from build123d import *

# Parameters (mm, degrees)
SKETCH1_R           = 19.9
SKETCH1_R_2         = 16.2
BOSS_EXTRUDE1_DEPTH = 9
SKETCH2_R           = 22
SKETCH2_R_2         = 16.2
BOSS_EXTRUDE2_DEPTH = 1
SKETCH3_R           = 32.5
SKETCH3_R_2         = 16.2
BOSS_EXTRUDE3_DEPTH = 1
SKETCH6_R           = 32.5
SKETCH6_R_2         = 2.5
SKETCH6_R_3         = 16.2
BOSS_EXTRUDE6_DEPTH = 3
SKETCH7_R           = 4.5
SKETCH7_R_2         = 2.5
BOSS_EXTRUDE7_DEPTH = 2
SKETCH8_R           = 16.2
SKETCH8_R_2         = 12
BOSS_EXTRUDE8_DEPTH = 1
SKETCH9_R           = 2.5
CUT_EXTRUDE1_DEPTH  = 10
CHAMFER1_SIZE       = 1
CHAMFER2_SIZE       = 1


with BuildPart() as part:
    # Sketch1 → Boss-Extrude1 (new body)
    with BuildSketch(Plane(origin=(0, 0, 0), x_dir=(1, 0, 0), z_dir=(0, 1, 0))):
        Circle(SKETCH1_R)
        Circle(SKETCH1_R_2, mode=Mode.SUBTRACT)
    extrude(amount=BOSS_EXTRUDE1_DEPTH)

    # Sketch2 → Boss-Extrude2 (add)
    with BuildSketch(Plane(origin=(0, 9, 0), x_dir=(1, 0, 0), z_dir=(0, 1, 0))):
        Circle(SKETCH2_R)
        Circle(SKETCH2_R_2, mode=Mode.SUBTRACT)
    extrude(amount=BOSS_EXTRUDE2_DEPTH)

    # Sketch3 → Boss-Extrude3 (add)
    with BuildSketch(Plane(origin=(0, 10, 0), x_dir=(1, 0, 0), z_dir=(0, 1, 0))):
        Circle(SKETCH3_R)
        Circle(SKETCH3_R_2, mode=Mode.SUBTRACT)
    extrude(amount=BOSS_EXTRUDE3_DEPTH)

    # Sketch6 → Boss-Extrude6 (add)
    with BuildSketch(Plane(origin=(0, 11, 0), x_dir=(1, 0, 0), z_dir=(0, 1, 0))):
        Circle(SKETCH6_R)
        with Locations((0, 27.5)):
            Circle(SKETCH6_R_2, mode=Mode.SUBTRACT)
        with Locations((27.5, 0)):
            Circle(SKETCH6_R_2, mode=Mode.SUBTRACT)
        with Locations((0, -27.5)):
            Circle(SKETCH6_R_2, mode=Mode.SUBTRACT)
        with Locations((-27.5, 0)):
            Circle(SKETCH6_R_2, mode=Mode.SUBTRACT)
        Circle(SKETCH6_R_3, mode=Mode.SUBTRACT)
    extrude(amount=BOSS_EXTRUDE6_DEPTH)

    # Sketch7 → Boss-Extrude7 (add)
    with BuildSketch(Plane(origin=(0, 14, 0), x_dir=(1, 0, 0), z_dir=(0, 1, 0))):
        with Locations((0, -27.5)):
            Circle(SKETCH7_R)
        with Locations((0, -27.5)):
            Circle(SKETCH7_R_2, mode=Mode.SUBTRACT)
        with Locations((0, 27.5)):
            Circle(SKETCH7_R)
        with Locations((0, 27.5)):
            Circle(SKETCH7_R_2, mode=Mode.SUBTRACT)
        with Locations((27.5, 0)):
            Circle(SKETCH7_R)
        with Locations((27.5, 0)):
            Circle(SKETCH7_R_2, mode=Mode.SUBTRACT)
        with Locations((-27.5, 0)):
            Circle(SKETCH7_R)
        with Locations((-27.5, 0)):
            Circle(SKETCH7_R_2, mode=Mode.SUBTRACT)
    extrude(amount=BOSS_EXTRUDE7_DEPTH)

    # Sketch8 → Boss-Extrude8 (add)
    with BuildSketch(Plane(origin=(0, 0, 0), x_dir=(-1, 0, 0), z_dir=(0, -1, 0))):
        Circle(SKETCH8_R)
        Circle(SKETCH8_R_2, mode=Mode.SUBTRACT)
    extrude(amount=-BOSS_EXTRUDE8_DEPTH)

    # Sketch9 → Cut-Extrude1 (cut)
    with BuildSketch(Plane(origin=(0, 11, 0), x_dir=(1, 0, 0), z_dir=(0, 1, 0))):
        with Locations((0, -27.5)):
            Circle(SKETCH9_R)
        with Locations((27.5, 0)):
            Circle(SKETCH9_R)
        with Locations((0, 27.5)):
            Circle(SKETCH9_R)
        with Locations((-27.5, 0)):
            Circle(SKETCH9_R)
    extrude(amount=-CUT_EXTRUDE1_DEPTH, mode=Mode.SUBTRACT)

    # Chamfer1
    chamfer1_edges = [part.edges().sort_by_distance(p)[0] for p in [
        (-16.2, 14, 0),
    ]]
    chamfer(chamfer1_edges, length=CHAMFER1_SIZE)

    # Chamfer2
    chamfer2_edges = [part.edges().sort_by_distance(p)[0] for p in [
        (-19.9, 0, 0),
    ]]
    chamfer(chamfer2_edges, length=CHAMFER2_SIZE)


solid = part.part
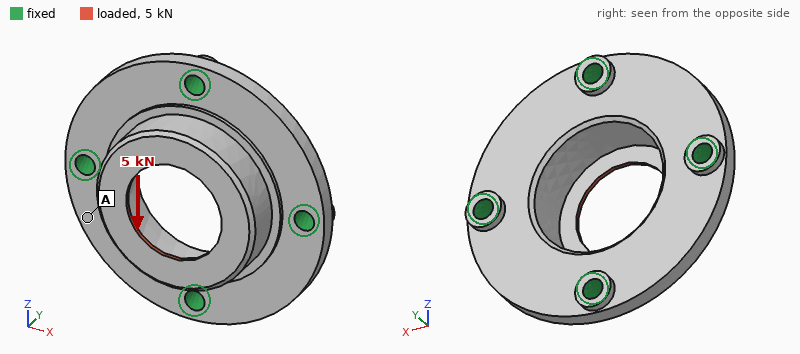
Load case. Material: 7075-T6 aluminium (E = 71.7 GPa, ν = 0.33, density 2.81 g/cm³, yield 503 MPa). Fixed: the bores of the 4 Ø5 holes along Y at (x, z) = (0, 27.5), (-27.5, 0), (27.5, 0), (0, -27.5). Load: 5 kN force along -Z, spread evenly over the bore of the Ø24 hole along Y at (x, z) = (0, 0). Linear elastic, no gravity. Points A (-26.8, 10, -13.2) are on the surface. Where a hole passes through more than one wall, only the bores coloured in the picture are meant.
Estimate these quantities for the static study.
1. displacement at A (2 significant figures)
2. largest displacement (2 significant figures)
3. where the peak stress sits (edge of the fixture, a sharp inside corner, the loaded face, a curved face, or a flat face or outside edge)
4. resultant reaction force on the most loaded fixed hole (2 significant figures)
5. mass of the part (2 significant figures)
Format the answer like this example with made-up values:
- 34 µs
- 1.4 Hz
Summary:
- 7.7 µm
- 40 µm
- the loaded face
- 1.7 kN
- 41 g
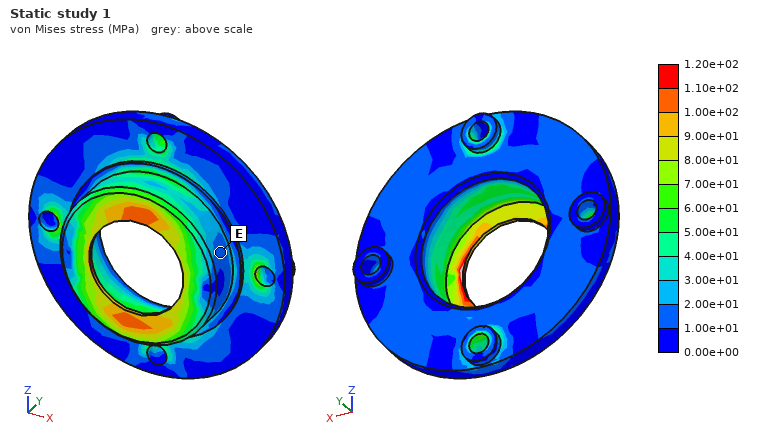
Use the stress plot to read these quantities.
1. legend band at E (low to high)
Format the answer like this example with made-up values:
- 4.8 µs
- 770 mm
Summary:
- 1.00e+01 to 2.00e+01 MPa
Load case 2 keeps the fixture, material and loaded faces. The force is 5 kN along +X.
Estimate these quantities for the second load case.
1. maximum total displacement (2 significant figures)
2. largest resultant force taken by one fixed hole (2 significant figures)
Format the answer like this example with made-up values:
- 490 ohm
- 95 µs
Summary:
- 40 µm
- 1.7 kN
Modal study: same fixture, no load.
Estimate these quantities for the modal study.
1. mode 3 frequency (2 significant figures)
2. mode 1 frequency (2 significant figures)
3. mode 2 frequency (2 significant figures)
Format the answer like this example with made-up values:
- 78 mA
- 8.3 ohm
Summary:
- 15 kHz
- 14 kHz
- 15 kHz
